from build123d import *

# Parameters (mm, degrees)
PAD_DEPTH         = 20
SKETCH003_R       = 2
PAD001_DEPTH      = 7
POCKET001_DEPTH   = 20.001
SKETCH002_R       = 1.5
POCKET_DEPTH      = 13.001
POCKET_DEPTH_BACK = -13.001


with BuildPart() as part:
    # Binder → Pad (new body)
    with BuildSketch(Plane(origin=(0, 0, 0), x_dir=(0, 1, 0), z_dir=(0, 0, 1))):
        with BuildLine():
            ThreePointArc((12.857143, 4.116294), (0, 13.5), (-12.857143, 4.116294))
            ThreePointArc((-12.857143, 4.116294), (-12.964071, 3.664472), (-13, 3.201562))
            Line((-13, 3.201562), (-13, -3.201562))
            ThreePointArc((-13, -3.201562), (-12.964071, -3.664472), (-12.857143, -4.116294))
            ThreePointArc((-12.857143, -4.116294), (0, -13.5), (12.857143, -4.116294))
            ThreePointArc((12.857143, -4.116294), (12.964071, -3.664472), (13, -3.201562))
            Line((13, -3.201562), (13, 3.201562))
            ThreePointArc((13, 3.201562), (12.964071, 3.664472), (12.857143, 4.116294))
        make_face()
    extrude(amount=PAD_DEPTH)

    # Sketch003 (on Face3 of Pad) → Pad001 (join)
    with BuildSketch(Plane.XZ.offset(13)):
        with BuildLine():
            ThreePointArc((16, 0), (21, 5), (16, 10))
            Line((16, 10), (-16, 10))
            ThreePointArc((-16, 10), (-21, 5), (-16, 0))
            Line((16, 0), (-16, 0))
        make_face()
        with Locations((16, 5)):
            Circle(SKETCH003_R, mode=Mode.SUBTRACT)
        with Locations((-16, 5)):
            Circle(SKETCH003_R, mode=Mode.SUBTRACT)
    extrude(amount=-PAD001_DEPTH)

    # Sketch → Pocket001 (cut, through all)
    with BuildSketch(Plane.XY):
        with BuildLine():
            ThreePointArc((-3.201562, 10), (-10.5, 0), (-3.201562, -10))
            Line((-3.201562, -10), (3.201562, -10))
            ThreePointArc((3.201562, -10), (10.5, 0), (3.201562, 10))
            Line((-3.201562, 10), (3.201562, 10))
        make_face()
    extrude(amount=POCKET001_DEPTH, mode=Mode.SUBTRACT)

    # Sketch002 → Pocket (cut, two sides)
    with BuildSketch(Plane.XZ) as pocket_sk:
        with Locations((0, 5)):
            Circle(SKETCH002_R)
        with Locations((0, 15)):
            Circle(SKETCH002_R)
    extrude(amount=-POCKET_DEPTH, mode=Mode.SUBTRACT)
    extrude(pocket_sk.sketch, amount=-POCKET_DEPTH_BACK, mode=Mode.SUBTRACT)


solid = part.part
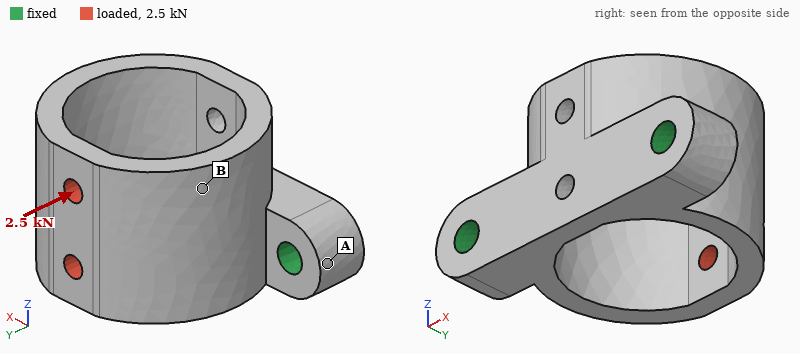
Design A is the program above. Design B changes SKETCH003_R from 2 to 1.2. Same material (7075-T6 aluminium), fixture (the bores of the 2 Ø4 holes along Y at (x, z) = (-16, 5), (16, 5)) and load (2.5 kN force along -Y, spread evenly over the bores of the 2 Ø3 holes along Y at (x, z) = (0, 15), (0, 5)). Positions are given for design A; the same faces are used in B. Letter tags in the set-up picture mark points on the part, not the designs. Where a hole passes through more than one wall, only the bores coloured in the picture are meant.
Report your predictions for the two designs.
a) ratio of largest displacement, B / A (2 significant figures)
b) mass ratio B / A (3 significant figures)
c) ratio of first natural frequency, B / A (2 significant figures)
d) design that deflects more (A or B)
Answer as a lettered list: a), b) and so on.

a) 1.1
b) 1.02
c) 0.91
d) B
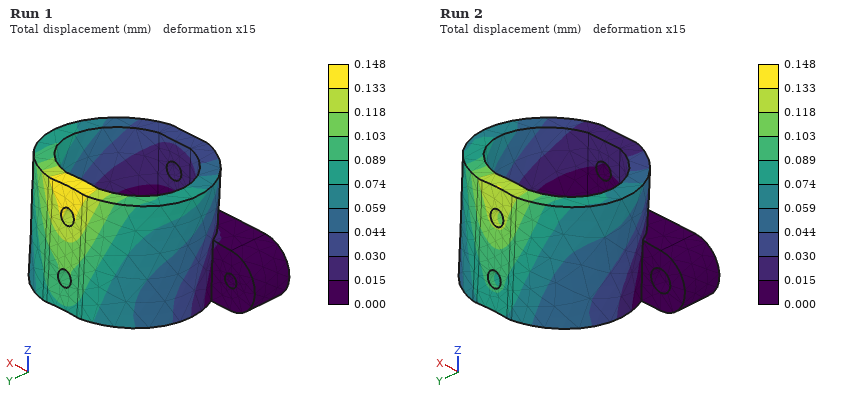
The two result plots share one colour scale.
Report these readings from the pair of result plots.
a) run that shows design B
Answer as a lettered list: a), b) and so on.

a) Run 1
